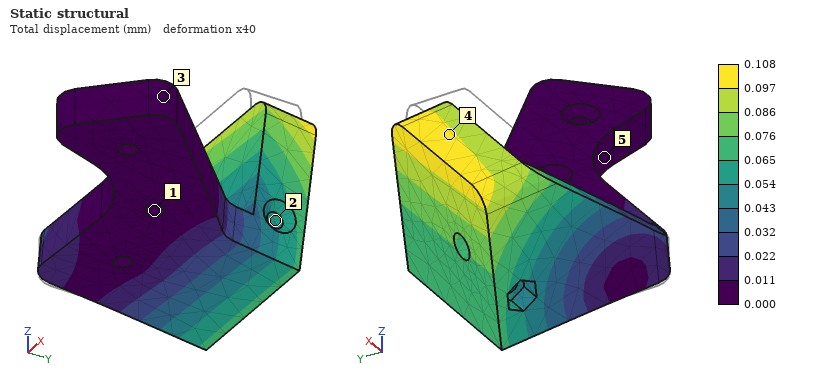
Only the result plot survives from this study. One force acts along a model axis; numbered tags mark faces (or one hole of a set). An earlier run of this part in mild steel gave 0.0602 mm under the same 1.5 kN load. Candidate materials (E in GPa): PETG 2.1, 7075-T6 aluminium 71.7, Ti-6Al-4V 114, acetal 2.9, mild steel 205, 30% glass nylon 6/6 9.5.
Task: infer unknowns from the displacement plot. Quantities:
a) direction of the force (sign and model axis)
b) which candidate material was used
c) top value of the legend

-Z
Ti-6Al-4V
0.108 mm
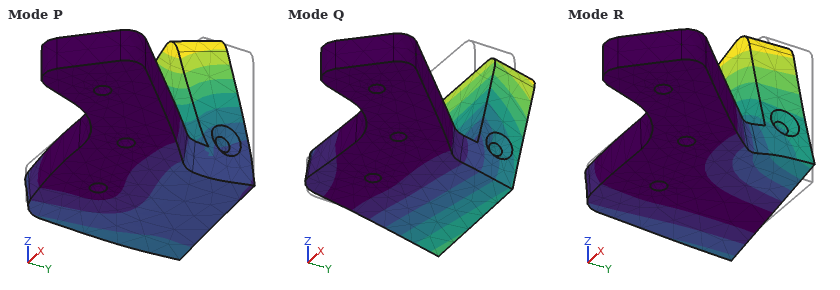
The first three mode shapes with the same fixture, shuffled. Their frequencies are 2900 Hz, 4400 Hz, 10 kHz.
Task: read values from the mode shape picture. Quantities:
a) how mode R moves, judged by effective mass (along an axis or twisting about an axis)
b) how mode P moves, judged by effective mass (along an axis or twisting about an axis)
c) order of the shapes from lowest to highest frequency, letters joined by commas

along X
along Z
Q, R, P
